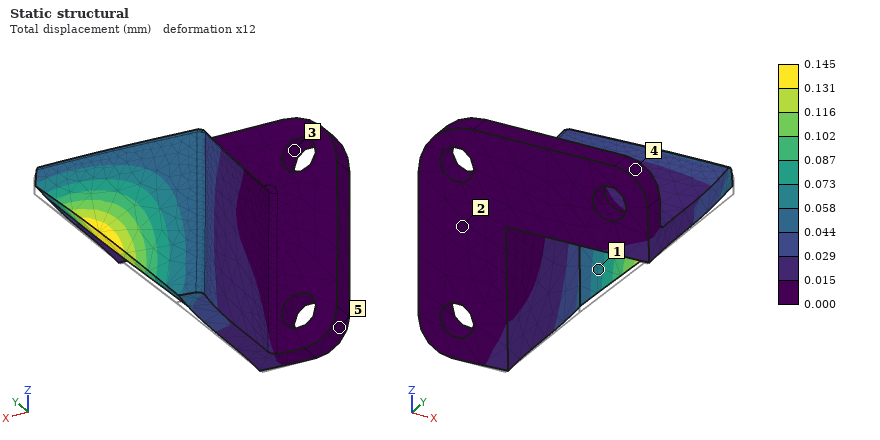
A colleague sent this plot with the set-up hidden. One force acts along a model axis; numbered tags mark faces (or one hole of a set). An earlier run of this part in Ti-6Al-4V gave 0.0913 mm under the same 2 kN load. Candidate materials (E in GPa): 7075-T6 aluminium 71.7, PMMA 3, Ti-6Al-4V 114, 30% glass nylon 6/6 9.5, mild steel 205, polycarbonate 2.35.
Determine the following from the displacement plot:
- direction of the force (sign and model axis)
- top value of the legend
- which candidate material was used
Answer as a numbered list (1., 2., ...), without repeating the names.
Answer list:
1. +Y
2. 0.145 mm
3. 7075-T6 aluminium
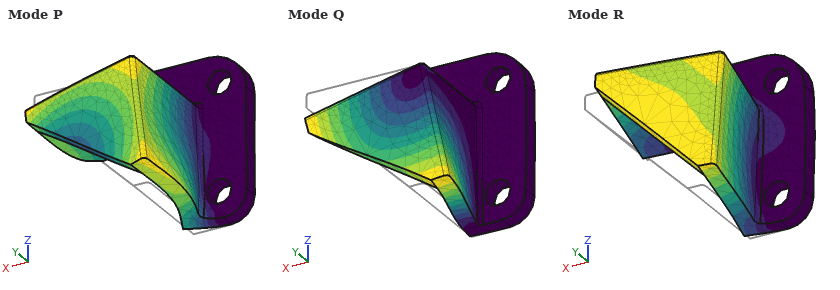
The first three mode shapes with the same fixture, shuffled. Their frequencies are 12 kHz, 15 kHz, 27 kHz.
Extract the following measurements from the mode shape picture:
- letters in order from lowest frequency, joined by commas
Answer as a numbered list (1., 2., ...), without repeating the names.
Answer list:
1. Q, R, P
